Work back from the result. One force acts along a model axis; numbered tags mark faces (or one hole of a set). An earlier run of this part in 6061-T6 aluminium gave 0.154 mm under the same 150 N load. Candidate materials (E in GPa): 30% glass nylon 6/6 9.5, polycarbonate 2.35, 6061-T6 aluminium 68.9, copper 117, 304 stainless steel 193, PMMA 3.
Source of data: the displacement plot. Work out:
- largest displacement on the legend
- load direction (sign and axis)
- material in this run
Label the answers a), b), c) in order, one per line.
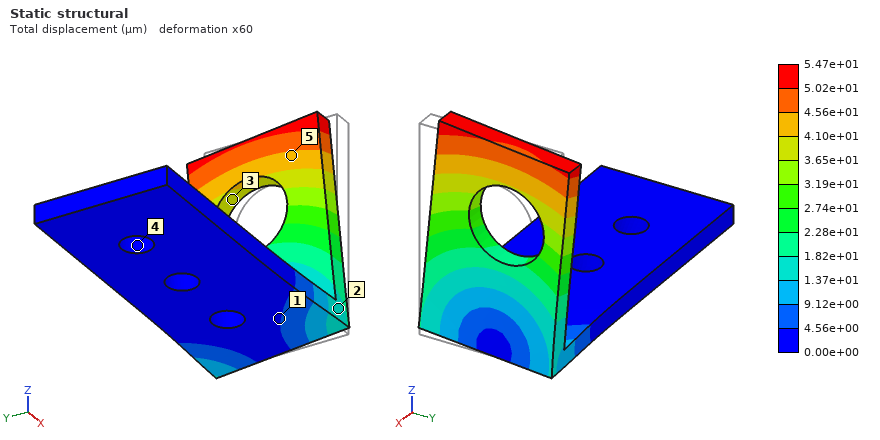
a) 5.47e+01 µm
b) +Y
c) 304 stainless steel
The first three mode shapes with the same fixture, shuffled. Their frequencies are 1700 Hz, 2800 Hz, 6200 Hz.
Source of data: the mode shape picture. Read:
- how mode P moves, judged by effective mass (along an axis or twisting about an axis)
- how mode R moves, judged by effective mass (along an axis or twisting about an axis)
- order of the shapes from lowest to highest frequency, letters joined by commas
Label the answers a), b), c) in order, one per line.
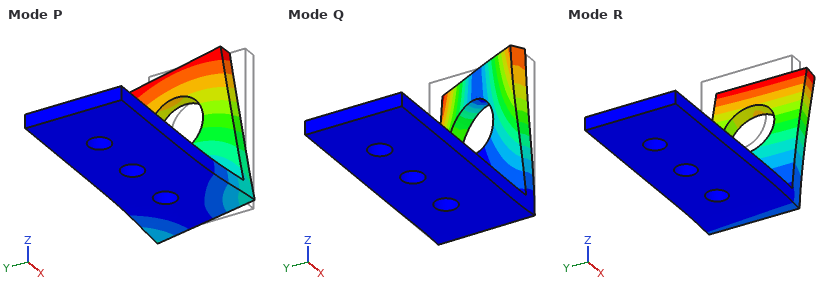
a) along Y
b) along X
c) R, P, Q
